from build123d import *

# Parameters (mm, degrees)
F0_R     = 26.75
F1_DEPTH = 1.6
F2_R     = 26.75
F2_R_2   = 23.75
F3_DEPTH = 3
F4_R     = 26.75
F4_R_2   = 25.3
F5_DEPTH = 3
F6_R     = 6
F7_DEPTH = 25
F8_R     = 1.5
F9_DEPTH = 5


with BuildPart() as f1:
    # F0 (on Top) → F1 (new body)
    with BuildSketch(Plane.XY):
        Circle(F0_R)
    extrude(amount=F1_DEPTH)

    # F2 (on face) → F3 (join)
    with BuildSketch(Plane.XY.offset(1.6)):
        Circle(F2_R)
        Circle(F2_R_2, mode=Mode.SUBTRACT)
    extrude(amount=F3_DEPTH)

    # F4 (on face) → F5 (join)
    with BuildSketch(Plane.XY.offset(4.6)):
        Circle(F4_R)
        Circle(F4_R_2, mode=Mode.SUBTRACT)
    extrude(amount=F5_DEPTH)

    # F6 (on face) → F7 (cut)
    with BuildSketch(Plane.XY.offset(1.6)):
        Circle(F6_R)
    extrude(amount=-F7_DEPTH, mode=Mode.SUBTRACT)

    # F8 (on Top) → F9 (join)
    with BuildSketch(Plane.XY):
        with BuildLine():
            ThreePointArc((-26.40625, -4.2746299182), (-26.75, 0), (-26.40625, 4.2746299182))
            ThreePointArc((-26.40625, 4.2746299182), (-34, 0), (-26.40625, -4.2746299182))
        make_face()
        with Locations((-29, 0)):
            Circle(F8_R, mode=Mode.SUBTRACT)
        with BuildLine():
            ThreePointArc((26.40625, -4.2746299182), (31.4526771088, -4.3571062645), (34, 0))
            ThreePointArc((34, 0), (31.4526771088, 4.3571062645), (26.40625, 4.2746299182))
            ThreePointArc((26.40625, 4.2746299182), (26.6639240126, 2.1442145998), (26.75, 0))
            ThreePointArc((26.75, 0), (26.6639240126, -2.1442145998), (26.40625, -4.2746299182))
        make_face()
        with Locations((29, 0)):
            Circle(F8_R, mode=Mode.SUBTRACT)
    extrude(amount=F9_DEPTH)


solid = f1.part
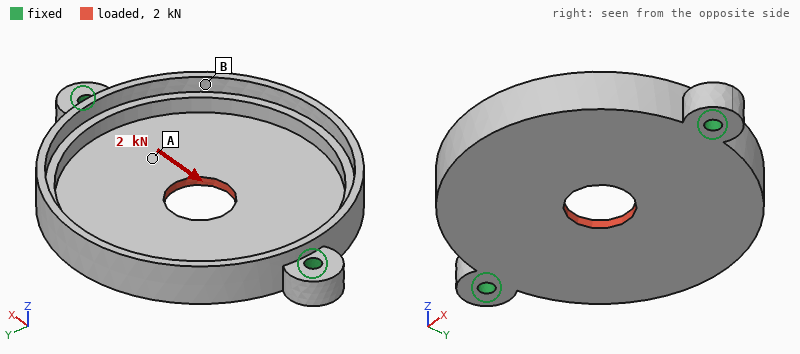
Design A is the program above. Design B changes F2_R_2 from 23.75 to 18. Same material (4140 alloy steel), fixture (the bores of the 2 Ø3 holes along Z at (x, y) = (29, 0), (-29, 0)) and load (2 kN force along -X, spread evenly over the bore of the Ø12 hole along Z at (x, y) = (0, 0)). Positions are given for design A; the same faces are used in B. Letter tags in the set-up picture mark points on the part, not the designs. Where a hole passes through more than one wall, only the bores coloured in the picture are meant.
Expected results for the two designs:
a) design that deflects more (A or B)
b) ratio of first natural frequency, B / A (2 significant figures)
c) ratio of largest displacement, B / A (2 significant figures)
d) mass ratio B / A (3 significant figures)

A
0.95
0.81
1.37
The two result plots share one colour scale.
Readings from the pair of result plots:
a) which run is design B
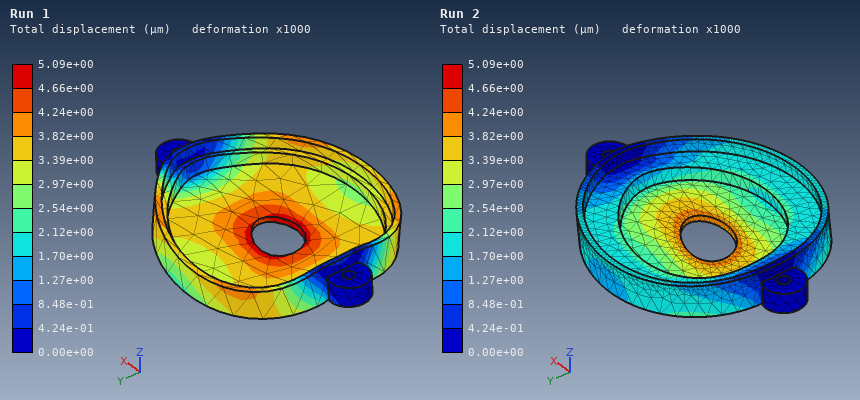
Run 2
